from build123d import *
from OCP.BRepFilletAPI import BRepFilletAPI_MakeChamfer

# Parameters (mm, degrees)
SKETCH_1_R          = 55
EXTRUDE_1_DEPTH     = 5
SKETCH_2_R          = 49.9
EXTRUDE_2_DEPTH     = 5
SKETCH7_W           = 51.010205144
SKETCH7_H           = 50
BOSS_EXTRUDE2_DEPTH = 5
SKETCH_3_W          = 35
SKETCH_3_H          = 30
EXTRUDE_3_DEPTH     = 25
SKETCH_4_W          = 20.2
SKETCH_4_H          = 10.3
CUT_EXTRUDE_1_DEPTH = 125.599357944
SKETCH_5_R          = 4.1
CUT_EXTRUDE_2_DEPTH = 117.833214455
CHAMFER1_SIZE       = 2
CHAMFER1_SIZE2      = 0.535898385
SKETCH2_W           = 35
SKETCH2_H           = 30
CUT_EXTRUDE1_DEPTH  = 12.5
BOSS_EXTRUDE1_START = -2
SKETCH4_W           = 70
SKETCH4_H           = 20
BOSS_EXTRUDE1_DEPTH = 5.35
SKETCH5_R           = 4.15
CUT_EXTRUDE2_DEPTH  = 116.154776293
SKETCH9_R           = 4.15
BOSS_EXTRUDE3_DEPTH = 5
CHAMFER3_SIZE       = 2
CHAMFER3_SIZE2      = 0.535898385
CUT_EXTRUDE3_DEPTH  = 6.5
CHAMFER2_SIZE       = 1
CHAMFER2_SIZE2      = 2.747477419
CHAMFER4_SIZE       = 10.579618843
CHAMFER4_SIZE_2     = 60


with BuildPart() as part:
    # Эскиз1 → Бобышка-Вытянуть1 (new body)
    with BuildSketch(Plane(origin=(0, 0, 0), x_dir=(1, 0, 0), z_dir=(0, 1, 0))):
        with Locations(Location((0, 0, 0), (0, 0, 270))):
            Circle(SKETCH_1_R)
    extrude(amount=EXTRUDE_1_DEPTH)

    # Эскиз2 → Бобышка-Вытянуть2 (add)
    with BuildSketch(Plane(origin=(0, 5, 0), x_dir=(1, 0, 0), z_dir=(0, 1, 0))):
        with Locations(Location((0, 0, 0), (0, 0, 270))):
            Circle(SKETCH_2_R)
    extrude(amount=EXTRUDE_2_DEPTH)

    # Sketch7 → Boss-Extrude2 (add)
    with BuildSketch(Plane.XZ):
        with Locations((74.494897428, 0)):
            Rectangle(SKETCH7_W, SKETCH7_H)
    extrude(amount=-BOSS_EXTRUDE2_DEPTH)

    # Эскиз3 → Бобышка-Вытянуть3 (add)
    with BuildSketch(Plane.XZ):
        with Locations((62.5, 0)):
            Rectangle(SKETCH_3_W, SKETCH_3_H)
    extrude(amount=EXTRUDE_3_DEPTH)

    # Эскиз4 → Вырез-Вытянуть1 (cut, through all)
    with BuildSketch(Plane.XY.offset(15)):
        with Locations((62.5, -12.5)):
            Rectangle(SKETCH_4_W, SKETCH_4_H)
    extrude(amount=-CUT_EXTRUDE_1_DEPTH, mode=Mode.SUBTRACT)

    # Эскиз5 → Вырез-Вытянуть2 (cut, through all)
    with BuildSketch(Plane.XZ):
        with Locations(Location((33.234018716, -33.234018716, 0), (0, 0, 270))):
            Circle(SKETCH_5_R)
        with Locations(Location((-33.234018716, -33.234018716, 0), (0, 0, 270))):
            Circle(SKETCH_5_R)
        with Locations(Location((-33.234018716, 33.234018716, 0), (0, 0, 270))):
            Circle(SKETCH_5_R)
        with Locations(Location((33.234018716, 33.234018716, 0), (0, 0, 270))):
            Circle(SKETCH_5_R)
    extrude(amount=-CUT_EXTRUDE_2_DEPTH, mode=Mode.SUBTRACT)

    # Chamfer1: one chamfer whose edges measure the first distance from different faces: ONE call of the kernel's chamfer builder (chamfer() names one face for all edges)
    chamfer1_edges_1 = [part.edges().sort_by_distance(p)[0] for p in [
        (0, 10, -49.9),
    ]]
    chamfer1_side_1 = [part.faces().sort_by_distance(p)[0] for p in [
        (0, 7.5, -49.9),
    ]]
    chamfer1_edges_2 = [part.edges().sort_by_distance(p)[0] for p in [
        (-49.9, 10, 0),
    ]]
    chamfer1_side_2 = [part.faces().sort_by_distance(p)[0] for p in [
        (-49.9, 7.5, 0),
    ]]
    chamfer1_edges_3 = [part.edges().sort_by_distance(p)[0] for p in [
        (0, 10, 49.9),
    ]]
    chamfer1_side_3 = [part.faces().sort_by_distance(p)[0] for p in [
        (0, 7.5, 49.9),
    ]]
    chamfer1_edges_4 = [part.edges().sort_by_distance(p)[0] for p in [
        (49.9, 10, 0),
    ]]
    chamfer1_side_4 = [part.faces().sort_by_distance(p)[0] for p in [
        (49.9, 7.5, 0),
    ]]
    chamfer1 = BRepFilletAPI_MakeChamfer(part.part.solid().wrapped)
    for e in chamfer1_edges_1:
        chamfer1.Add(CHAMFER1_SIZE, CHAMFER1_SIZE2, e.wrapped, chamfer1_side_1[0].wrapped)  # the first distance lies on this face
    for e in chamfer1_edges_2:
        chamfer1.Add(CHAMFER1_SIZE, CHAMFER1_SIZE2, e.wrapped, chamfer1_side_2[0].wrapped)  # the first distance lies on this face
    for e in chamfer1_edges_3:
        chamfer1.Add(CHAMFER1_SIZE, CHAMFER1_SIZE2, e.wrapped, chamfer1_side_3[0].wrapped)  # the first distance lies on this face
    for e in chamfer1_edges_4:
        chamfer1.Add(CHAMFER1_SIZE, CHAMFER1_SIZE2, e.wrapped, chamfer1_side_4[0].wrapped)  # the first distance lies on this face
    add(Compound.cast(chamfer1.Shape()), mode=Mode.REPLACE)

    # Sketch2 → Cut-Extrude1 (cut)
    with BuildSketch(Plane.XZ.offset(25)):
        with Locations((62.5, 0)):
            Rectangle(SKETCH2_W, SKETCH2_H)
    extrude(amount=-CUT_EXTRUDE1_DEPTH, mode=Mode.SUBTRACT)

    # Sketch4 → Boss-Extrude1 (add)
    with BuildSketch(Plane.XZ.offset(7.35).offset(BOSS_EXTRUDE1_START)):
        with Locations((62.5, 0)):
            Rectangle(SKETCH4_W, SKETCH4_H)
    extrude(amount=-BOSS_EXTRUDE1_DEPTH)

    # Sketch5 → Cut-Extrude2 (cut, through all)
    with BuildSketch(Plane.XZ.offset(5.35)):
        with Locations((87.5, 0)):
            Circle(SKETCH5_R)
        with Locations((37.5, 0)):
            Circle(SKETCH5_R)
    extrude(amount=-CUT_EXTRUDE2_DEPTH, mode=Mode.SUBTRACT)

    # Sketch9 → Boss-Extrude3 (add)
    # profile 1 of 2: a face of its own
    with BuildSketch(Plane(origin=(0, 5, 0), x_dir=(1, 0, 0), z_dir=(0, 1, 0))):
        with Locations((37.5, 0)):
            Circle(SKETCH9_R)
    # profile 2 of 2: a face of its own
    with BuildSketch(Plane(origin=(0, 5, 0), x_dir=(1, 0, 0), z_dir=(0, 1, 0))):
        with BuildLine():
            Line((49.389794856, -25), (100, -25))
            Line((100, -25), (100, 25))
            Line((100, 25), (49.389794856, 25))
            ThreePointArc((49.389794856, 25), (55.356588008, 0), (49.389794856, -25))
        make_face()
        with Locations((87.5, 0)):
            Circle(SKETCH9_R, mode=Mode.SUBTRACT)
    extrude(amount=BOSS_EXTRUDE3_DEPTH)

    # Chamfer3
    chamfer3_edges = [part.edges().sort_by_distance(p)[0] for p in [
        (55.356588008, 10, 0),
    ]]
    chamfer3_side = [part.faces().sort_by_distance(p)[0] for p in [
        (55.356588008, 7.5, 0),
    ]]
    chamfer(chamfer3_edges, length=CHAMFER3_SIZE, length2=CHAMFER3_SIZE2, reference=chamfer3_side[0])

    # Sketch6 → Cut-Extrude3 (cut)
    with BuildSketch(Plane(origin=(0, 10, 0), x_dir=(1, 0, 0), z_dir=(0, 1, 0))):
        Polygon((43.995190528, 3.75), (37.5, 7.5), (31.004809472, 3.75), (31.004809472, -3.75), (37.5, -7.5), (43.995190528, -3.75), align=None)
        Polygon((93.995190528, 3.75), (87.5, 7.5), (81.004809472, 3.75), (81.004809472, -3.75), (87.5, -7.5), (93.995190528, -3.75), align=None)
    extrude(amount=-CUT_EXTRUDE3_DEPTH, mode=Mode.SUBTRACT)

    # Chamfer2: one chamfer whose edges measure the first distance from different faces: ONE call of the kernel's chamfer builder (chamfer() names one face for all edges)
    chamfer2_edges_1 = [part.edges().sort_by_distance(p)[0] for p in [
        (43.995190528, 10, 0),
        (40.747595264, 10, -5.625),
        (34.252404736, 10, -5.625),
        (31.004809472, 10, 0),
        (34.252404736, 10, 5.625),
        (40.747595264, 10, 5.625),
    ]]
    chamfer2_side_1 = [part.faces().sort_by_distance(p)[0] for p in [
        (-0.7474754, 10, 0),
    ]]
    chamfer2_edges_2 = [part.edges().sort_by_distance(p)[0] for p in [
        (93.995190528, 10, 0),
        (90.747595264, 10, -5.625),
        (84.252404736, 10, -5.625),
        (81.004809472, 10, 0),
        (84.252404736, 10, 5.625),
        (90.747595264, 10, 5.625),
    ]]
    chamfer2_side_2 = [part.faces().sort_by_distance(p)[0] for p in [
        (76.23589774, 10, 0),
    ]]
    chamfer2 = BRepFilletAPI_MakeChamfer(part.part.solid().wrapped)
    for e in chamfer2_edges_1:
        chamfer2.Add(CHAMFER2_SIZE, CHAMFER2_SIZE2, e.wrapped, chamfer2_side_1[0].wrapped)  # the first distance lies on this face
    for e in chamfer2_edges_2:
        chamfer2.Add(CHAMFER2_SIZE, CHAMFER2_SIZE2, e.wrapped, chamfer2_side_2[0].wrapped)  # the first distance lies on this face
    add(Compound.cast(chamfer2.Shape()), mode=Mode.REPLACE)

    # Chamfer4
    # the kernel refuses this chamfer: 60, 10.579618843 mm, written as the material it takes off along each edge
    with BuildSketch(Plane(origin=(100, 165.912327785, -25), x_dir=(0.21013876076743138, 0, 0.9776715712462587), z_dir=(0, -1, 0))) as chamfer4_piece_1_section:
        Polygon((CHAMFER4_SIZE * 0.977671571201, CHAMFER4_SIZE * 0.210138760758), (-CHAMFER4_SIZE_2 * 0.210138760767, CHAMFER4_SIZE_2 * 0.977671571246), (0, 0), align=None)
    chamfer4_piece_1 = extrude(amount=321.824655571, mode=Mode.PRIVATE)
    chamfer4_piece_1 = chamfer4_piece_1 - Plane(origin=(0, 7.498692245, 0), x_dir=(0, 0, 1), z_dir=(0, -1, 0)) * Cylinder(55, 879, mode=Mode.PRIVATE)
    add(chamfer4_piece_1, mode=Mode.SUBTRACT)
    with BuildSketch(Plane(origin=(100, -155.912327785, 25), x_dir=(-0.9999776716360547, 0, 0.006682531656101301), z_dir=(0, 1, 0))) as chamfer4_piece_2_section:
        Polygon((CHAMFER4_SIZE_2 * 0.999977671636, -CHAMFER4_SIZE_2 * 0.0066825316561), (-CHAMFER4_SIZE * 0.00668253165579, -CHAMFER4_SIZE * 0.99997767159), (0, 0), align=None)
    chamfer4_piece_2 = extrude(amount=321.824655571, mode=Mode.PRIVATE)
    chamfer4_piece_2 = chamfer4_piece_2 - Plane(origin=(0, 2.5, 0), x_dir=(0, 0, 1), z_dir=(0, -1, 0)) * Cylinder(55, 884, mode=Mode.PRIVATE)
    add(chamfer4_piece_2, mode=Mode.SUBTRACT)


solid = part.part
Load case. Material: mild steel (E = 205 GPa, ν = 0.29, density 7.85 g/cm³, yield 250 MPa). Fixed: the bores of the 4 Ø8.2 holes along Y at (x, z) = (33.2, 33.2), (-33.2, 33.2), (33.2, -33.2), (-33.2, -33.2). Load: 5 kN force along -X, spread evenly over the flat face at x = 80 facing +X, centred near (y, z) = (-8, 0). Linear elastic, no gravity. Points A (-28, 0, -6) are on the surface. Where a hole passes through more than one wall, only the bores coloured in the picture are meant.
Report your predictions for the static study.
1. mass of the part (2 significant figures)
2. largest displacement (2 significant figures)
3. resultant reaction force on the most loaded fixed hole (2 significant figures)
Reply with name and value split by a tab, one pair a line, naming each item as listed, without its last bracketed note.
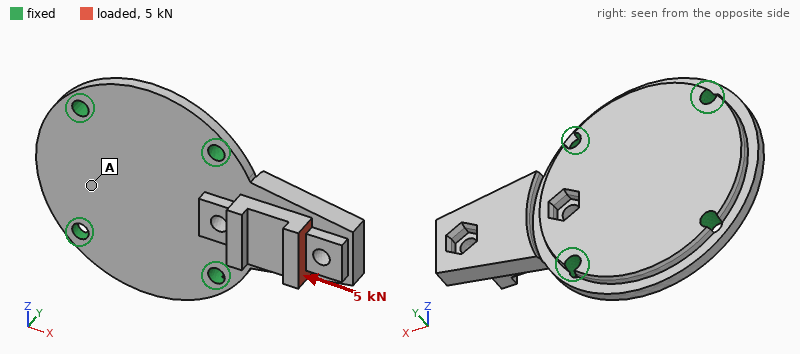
mass of the part	880 g
largest displacement	0.11 mm
resultant reaction force on the most loaded fixed hole	1.7 kN
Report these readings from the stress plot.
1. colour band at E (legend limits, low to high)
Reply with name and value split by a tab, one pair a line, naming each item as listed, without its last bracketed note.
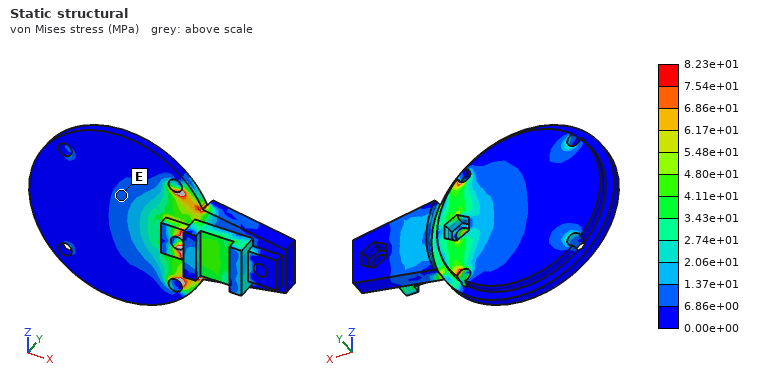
colour band at E	6.86e+00 to 1.37e+01 MPa
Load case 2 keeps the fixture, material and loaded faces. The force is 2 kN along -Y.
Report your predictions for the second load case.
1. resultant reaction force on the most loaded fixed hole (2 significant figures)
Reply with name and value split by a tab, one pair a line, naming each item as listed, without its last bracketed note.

resultant reaction force on the most loaded fixed hole	1.6 kN
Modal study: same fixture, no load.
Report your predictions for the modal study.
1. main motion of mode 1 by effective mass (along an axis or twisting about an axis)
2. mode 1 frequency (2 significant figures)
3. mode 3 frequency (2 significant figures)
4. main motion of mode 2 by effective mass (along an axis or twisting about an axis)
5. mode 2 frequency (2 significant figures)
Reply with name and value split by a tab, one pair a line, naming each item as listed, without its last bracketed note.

main motion of mode 1 by effective mass	along Y
mode 1 frequency	1700 Hz
mode 3 frequency	7800 Hz
main motion of mode 2 by effective mass	along Z
mode 2 frequency	6800 Hz
